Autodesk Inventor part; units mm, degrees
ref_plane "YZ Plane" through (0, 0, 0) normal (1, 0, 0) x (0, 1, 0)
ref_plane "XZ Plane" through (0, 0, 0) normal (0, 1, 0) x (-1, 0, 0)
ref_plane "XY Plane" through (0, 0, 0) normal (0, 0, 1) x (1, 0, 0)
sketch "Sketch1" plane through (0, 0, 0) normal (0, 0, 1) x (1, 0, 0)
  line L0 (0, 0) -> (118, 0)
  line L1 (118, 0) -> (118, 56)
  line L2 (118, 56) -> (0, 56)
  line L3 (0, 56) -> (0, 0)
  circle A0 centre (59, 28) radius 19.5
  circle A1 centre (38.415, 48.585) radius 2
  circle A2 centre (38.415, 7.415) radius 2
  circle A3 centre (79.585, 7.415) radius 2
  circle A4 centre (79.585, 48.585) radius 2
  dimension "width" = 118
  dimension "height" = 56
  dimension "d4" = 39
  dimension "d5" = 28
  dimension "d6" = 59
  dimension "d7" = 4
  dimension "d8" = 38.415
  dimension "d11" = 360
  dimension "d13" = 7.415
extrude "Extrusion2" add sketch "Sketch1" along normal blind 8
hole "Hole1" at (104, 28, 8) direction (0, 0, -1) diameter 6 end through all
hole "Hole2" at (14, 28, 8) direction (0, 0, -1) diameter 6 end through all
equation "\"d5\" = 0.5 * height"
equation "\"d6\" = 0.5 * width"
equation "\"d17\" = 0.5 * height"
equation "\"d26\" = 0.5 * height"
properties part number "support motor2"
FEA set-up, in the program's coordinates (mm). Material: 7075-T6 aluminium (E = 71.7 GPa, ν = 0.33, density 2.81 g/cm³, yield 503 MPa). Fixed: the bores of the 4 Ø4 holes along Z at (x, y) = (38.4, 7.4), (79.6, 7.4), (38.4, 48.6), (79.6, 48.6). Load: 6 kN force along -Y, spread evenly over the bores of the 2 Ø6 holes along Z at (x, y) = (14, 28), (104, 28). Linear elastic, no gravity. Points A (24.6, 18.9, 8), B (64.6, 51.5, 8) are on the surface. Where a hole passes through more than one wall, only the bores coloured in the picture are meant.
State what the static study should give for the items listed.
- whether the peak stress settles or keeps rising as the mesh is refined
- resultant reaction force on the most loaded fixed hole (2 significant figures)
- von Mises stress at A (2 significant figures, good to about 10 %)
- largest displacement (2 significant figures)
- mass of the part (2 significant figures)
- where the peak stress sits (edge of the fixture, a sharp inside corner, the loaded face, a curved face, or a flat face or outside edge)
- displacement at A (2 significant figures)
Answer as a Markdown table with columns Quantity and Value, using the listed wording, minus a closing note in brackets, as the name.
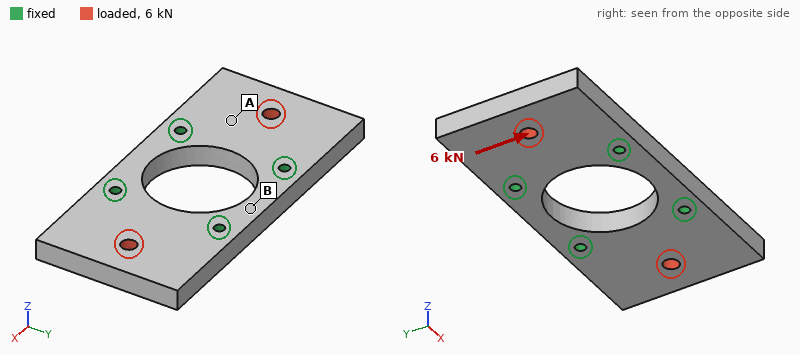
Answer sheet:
| Quantity | Value |
|---|---|
| whether the peak stress settles or keeps rising as the mesh is refined | keeps rising |
| resultant reaction force on the most loaded fixed hole | 2.1 kN |
| von Mises stress at A | 16 MPa |
| largest displacement | 13 µm |
| mass of the part | 120 g |
| where the peak stress sits | edge of the fixture |
| displacement at A | 5.7 µm |
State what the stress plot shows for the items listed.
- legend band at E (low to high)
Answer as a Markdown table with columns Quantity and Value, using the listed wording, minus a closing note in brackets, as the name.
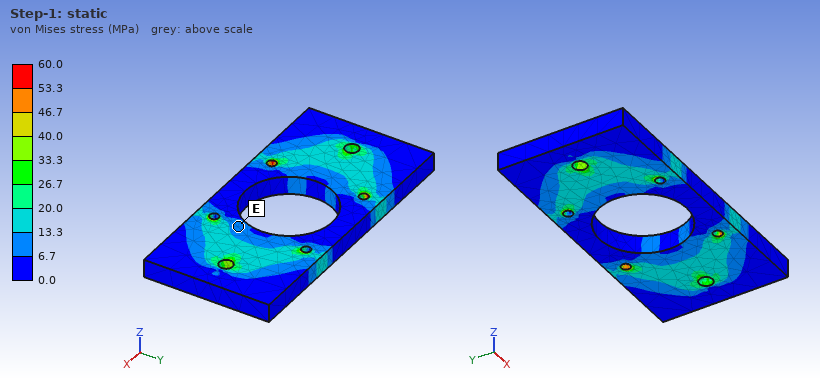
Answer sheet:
| Quantity | Value |
|---|---|
| legend band at E | 6.7 to 13.3 MPa |
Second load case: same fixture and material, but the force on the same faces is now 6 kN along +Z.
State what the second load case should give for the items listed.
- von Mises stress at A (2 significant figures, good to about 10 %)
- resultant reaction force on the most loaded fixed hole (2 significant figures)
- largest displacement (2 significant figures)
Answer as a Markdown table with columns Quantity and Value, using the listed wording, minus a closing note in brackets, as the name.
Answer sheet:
| Quantity | Value |
|---|---|
| von Mises stress at A | 57 MPa |
| resultant reaction force on the most loaded fixed hole | 1.5 kN |
| largest displacement | 0.28 mm |
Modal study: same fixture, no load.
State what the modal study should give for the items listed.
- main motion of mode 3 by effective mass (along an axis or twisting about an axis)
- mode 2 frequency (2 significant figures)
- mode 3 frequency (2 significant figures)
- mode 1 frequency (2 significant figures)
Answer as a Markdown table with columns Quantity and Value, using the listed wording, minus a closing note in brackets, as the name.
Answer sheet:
| Quantity | Value |
|---|---|
| main motion of mode 3 by effective mass | twisting about X |
| mode 2 frequency | 3600 Hz |
| mode 3 frequency | 7400 Hz |
| mode 1 frequency | 3600 Hz |
